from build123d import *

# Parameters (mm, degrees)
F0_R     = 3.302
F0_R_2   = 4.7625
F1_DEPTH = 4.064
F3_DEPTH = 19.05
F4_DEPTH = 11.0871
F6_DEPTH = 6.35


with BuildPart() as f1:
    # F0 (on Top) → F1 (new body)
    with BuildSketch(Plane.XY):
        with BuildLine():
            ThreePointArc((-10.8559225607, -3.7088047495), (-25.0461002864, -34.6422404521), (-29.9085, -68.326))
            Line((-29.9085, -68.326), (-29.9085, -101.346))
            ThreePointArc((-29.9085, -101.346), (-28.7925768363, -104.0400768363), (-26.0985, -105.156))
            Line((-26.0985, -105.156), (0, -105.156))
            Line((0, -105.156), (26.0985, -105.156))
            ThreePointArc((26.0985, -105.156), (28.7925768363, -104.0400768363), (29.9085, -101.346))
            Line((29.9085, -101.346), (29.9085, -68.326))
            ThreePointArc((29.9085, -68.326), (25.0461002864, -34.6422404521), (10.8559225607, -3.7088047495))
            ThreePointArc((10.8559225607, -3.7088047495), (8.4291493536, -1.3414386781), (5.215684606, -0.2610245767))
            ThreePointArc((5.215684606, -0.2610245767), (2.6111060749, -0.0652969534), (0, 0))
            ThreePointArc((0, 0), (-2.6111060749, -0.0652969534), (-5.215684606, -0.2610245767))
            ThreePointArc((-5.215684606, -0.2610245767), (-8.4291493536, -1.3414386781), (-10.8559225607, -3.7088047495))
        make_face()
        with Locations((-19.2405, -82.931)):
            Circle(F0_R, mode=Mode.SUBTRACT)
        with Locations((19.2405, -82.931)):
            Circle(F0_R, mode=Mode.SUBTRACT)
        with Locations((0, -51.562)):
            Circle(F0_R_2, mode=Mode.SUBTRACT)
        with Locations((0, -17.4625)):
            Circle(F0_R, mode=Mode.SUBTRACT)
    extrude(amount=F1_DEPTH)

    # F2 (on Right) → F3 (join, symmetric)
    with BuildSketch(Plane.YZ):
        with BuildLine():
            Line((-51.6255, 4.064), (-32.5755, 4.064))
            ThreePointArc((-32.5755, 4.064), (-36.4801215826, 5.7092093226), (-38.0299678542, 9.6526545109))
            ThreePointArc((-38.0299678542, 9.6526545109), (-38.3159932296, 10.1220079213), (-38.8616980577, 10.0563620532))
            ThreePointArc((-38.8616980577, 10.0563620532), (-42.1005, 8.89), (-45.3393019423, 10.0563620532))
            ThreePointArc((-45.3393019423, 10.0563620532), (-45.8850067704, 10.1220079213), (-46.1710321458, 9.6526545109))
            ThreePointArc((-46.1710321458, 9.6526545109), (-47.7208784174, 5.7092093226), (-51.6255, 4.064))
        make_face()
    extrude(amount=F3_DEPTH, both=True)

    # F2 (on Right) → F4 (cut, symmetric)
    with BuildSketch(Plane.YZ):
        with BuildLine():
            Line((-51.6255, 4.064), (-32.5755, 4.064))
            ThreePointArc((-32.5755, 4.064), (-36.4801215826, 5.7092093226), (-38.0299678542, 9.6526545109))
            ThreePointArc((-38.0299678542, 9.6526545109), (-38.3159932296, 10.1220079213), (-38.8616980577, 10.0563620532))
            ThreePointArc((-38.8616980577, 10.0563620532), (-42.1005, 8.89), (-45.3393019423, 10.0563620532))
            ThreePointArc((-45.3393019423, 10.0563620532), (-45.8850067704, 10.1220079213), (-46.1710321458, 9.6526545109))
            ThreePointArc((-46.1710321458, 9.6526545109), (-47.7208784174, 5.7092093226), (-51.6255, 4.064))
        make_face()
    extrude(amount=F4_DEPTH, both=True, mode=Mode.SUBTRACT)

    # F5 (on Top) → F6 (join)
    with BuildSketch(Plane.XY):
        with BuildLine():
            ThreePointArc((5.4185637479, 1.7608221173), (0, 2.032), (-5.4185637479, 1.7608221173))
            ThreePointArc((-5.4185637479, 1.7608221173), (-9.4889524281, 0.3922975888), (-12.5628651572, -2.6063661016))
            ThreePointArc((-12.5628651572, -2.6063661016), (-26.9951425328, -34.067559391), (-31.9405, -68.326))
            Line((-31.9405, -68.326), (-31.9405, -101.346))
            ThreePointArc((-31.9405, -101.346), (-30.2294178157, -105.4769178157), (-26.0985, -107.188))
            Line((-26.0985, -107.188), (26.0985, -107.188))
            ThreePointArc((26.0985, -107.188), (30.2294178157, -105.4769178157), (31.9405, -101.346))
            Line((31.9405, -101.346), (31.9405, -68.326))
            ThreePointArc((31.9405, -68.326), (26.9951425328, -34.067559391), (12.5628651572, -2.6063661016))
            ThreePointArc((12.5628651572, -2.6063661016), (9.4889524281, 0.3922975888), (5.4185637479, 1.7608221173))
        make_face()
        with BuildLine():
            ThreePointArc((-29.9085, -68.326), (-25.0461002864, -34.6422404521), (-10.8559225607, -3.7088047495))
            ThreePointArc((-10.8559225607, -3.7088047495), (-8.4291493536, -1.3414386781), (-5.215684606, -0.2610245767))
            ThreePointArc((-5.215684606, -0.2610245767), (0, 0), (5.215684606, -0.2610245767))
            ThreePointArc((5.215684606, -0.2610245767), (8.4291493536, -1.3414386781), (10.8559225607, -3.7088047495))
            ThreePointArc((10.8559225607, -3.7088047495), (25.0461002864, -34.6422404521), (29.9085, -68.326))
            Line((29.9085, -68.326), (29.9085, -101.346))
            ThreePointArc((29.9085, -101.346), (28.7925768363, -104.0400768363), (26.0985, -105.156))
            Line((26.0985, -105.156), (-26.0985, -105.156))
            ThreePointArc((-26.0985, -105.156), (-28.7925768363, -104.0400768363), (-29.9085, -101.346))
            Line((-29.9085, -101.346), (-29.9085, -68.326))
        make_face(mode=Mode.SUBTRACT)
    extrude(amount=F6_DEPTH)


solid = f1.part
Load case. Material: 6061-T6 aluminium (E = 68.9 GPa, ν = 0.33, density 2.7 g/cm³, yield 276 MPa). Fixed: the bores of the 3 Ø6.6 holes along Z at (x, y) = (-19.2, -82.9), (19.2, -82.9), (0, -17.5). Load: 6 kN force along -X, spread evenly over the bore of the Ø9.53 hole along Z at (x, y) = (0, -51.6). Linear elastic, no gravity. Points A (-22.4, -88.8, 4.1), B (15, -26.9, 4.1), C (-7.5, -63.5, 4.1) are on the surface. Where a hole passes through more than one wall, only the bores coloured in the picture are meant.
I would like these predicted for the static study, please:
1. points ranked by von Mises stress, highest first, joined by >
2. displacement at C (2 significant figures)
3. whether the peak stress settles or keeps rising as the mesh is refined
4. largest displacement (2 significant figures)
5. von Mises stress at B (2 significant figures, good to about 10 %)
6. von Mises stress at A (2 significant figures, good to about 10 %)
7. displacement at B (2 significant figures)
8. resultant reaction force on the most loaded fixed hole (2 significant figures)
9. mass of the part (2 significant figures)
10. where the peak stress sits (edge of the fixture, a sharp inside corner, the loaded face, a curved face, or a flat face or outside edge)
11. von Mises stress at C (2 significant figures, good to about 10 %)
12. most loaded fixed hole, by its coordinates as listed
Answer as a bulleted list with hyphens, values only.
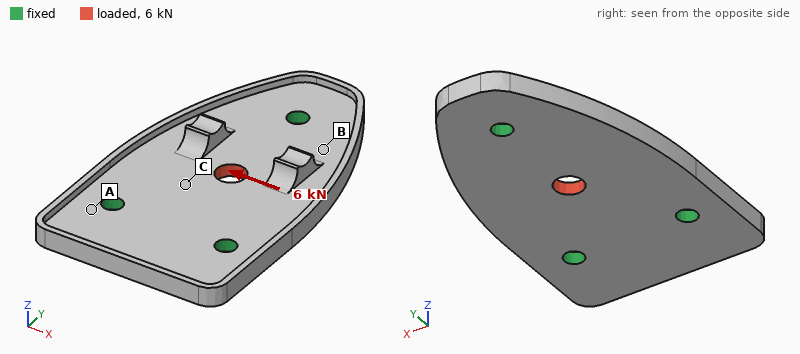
- C > B > A
- 14 µm
- keeps rising
- 26 µm
- 23 MPa
- 11 MPa
- 10 µm
- 2.3 kN
- 69 g
- edge of the fixture
- 37 MPa
- (0, -17.5)
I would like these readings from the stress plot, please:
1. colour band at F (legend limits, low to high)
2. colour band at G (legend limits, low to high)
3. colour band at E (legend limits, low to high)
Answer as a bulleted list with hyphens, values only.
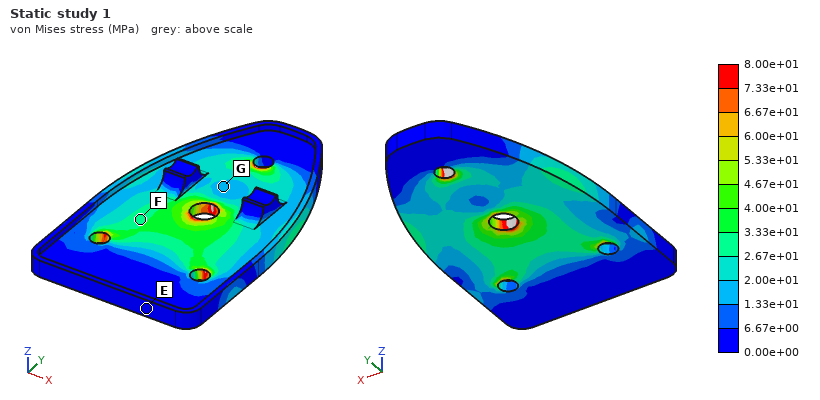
- 2.67e+01 to 3.33e+01 MPa
- 1.33e+01 to 2.00e+01 MPa
- 0.00e+00 to 6.67e+00 MPa
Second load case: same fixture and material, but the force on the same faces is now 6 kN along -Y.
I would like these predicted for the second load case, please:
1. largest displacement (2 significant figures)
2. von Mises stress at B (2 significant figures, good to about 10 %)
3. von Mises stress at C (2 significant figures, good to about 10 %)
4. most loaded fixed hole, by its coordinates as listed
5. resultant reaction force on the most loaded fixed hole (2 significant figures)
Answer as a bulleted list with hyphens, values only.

- 14 µm
- 8.5 MPa
- 27 MPa
- (0, -17.5)
- 2.4 kN
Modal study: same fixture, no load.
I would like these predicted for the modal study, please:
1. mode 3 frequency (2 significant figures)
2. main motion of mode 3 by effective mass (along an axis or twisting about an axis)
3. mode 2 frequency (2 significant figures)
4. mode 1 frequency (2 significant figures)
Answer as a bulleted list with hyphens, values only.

- 5700 Hz
- along Z
- 4300 Hz
- 4300 Hz
